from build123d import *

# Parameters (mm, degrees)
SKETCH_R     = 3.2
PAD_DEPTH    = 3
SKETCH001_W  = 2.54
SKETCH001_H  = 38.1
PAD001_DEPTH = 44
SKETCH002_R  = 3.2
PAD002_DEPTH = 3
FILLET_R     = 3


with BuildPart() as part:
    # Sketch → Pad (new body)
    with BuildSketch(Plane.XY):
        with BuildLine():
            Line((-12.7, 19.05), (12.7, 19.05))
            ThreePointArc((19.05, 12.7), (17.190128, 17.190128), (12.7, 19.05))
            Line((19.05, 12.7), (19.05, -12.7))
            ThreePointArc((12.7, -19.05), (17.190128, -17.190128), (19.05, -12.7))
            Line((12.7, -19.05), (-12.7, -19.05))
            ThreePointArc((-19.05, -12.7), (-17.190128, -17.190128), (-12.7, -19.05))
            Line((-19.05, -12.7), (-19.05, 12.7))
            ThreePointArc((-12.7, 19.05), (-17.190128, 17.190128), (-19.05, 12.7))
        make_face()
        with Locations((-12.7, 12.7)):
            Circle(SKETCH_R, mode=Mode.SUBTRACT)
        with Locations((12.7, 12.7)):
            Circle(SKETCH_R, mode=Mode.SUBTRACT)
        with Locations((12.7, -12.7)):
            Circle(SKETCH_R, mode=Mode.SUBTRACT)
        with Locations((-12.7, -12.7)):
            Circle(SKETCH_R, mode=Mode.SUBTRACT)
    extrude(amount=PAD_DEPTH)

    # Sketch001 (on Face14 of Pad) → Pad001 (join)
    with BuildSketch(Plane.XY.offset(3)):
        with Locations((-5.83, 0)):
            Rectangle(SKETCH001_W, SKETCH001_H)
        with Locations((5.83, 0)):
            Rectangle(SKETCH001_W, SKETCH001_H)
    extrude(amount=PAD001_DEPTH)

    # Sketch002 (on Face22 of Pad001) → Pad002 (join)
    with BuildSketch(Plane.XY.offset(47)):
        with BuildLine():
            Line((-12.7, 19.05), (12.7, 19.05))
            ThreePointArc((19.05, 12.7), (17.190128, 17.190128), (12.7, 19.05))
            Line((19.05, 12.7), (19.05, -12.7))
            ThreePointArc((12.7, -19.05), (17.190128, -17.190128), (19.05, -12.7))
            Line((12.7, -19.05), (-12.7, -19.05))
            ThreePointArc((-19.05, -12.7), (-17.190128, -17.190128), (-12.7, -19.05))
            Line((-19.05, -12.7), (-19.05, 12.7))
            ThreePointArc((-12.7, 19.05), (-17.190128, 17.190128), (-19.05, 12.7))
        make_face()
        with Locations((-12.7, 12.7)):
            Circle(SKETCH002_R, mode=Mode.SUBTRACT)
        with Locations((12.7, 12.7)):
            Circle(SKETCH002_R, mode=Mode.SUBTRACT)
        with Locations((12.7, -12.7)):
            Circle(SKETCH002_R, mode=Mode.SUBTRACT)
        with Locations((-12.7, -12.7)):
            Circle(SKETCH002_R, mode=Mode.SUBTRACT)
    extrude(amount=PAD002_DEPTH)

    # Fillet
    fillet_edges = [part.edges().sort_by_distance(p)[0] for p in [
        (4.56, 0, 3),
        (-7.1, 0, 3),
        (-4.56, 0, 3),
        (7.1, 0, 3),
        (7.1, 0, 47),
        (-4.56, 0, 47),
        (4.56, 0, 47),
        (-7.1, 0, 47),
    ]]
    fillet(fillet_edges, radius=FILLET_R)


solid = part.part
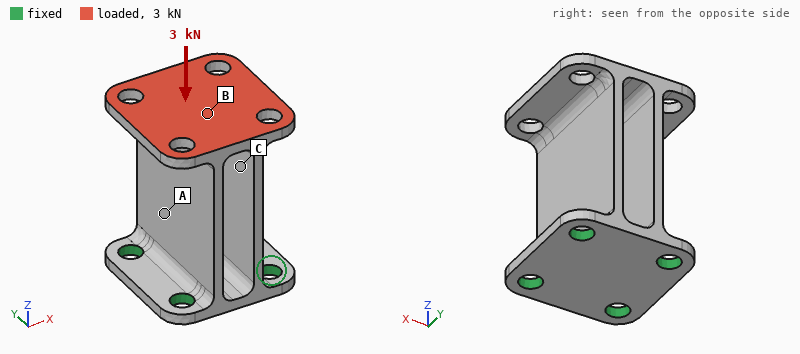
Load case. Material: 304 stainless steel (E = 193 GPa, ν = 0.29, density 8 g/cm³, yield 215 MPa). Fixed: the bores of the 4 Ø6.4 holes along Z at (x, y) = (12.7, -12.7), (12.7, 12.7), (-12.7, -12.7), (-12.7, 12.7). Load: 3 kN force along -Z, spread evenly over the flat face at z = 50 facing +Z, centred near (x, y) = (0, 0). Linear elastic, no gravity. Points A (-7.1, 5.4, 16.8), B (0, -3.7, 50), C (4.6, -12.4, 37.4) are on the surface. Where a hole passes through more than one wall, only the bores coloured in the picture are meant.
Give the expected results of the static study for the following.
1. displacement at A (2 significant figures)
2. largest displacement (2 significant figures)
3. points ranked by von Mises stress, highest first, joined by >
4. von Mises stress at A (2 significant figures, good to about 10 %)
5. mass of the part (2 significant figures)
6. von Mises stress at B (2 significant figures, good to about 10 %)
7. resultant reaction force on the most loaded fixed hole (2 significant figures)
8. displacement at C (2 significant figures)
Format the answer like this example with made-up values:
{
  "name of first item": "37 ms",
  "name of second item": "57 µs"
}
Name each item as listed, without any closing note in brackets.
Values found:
{
  "displacement at A": "8.5 µm",
  "largest displacement": "34 µm",
  "points ranked by von Mises stress, highest first, joined by >": "B > A > C",
  "von Mises stress at A": "20 MPa",
  "mass of the part": "130 g",
  "von Mises stress at B": "67 MPa",
  "resultant reaction force on the most loaded fixed hole": "770 N",
  "displacement at C": "10 µm"
}
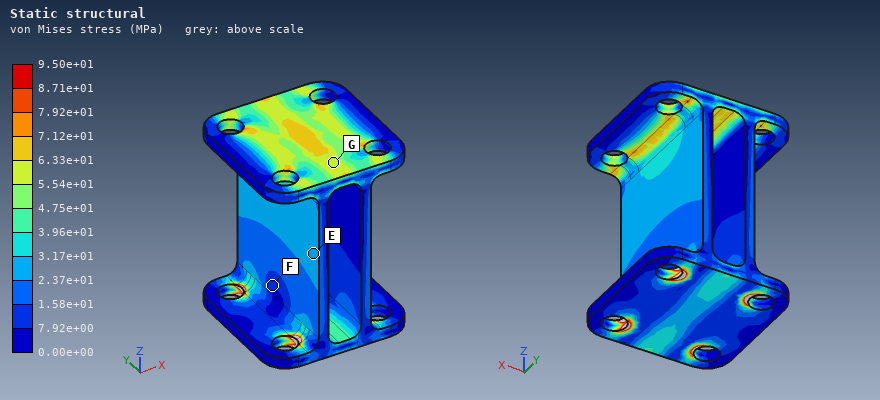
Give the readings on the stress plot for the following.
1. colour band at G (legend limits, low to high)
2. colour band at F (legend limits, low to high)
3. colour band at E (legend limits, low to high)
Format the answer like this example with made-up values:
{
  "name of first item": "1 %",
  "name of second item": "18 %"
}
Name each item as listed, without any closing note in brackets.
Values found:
{
  "colour band at G": "5.54e+01 to 6.33e+01 MPa",
  "colour band at F": "7.92e+00 to 1.58e+01 MPa",
  "colour band at E": "2.37e+01 to 3.17e+01 MPa"
}
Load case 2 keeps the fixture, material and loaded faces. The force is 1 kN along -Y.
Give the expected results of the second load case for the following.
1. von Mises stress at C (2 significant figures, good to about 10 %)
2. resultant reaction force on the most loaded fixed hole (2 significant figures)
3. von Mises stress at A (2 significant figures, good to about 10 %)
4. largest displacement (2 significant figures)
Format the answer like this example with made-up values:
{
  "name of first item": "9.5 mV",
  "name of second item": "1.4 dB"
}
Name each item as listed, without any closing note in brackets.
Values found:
{
  "von Mises stress at C": "14 MPa",
  "resultant reaction force on the most loaded fixed hole": "940 N",
  "von Mises stress at A": "15 MPa",
  "largest displacement": "26 µm"
}
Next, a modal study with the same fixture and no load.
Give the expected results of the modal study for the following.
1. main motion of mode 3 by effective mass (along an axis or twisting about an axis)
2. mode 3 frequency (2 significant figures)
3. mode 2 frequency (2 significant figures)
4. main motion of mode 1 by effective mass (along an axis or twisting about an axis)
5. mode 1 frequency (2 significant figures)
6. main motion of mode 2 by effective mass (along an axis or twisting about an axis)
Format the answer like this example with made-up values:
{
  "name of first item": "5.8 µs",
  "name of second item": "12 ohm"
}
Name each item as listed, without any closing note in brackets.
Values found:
{
  "main motion of mode 3 by effective mass": "along Y",
  "mode 3 frequency": "4400 Hz",
  "mode 2 frequency": "3000 Hz",
  "main motion of mode 1 by effective mass": "along X",
  "mode 1 frequency": "1200 Hz",
  "main motion of mode 2 by effective mass": "twisting about Z"
}
